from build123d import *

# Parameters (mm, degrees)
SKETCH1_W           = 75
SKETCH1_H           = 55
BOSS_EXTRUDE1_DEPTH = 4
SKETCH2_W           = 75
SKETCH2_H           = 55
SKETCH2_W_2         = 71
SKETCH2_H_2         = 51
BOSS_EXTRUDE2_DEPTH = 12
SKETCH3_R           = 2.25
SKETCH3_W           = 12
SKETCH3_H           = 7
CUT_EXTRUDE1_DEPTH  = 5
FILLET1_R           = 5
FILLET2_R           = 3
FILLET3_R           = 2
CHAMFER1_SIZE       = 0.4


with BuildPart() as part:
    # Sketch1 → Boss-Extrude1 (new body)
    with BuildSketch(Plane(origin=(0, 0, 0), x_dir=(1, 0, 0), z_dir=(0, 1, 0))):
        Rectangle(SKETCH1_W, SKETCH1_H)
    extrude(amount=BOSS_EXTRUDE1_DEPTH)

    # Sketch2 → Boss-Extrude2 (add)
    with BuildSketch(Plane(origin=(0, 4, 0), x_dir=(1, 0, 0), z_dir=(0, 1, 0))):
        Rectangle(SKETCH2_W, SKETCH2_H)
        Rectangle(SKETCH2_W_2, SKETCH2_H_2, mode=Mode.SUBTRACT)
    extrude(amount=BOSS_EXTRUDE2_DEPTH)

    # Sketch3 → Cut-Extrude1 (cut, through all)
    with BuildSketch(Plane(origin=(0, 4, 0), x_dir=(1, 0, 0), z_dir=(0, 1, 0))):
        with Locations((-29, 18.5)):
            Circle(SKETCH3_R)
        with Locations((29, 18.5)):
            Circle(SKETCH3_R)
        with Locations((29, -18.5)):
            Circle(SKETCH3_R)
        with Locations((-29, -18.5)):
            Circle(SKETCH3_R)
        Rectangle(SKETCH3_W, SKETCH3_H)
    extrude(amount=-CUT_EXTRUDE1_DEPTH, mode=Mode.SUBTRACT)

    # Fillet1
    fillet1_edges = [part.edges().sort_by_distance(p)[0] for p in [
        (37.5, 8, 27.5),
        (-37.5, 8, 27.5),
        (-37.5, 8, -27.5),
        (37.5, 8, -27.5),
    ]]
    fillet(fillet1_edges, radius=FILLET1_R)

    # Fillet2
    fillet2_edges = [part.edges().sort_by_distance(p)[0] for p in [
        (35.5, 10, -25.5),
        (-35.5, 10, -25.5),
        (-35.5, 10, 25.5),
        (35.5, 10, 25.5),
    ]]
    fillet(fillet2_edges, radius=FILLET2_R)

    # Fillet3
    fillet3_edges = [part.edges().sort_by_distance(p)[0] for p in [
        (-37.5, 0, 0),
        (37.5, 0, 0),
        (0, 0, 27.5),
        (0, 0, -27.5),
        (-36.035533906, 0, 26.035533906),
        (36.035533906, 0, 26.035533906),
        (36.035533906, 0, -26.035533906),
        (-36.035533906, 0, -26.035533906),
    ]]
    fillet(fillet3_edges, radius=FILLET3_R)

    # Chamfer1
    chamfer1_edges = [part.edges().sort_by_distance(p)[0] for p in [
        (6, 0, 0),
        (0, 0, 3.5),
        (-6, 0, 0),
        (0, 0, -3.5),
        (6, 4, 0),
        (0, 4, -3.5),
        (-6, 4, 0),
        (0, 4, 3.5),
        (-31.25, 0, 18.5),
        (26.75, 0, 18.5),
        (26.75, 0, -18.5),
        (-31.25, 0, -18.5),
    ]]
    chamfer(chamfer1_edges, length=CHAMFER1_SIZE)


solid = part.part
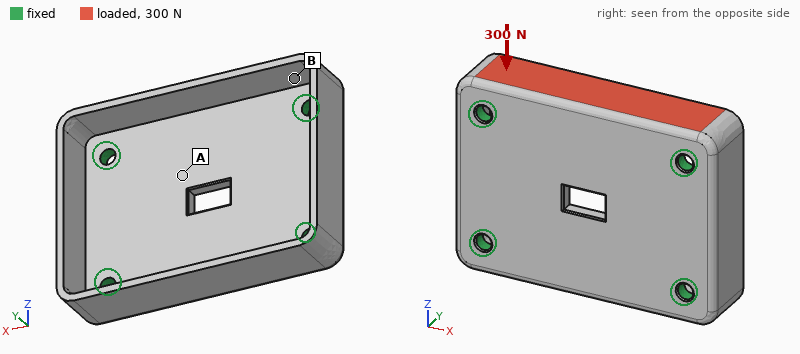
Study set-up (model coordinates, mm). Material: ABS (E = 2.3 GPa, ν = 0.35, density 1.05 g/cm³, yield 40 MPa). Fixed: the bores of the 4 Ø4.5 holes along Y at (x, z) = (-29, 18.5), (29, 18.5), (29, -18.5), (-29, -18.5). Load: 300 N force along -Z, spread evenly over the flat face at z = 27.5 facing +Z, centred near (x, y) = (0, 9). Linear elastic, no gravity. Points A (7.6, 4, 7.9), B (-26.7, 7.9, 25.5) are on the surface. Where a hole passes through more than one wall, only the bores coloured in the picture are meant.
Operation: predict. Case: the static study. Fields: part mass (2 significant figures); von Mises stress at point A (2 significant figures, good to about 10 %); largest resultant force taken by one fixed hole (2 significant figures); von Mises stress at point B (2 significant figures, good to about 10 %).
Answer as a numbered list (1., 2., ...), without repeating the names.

1. 23 g
2. 4.4 MPa
3. 90 N
4. 9.7 MPa
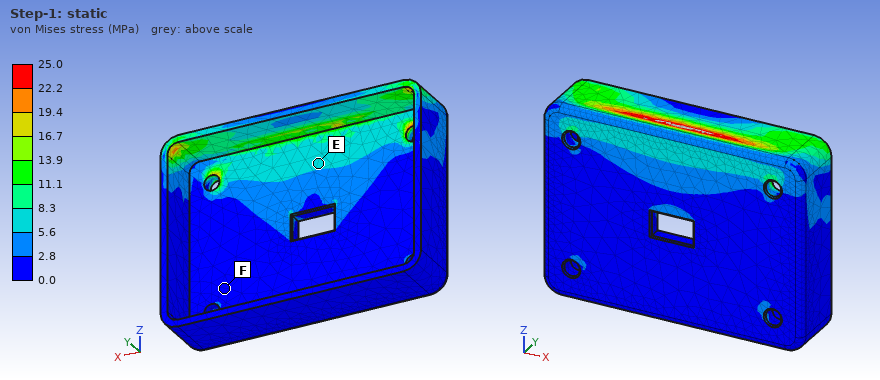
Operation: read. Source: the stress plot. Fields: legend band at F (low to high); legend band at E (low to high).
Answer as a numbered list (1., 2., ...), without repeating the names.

1. 0.0 to 2.8 MPa
2. 5.6 to 8.3 MPa
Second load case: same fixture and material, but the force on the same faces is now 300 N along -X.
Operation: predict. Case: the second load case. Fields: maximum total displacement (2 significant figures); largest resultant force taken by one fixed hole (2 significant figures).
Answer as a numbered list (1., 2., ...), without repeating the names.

1. 49 µm
2. 150 N
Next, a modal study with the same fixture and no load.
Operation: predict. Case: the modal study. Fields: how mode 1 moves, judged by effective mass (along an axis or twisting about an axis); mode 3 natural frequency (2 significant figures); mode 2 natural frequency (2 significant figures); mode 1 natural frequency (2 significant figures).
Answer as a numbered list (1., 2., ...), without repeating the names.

1. along Y
2. 2500 Hz
3. 2500 Hz
4. 1900 Hz
